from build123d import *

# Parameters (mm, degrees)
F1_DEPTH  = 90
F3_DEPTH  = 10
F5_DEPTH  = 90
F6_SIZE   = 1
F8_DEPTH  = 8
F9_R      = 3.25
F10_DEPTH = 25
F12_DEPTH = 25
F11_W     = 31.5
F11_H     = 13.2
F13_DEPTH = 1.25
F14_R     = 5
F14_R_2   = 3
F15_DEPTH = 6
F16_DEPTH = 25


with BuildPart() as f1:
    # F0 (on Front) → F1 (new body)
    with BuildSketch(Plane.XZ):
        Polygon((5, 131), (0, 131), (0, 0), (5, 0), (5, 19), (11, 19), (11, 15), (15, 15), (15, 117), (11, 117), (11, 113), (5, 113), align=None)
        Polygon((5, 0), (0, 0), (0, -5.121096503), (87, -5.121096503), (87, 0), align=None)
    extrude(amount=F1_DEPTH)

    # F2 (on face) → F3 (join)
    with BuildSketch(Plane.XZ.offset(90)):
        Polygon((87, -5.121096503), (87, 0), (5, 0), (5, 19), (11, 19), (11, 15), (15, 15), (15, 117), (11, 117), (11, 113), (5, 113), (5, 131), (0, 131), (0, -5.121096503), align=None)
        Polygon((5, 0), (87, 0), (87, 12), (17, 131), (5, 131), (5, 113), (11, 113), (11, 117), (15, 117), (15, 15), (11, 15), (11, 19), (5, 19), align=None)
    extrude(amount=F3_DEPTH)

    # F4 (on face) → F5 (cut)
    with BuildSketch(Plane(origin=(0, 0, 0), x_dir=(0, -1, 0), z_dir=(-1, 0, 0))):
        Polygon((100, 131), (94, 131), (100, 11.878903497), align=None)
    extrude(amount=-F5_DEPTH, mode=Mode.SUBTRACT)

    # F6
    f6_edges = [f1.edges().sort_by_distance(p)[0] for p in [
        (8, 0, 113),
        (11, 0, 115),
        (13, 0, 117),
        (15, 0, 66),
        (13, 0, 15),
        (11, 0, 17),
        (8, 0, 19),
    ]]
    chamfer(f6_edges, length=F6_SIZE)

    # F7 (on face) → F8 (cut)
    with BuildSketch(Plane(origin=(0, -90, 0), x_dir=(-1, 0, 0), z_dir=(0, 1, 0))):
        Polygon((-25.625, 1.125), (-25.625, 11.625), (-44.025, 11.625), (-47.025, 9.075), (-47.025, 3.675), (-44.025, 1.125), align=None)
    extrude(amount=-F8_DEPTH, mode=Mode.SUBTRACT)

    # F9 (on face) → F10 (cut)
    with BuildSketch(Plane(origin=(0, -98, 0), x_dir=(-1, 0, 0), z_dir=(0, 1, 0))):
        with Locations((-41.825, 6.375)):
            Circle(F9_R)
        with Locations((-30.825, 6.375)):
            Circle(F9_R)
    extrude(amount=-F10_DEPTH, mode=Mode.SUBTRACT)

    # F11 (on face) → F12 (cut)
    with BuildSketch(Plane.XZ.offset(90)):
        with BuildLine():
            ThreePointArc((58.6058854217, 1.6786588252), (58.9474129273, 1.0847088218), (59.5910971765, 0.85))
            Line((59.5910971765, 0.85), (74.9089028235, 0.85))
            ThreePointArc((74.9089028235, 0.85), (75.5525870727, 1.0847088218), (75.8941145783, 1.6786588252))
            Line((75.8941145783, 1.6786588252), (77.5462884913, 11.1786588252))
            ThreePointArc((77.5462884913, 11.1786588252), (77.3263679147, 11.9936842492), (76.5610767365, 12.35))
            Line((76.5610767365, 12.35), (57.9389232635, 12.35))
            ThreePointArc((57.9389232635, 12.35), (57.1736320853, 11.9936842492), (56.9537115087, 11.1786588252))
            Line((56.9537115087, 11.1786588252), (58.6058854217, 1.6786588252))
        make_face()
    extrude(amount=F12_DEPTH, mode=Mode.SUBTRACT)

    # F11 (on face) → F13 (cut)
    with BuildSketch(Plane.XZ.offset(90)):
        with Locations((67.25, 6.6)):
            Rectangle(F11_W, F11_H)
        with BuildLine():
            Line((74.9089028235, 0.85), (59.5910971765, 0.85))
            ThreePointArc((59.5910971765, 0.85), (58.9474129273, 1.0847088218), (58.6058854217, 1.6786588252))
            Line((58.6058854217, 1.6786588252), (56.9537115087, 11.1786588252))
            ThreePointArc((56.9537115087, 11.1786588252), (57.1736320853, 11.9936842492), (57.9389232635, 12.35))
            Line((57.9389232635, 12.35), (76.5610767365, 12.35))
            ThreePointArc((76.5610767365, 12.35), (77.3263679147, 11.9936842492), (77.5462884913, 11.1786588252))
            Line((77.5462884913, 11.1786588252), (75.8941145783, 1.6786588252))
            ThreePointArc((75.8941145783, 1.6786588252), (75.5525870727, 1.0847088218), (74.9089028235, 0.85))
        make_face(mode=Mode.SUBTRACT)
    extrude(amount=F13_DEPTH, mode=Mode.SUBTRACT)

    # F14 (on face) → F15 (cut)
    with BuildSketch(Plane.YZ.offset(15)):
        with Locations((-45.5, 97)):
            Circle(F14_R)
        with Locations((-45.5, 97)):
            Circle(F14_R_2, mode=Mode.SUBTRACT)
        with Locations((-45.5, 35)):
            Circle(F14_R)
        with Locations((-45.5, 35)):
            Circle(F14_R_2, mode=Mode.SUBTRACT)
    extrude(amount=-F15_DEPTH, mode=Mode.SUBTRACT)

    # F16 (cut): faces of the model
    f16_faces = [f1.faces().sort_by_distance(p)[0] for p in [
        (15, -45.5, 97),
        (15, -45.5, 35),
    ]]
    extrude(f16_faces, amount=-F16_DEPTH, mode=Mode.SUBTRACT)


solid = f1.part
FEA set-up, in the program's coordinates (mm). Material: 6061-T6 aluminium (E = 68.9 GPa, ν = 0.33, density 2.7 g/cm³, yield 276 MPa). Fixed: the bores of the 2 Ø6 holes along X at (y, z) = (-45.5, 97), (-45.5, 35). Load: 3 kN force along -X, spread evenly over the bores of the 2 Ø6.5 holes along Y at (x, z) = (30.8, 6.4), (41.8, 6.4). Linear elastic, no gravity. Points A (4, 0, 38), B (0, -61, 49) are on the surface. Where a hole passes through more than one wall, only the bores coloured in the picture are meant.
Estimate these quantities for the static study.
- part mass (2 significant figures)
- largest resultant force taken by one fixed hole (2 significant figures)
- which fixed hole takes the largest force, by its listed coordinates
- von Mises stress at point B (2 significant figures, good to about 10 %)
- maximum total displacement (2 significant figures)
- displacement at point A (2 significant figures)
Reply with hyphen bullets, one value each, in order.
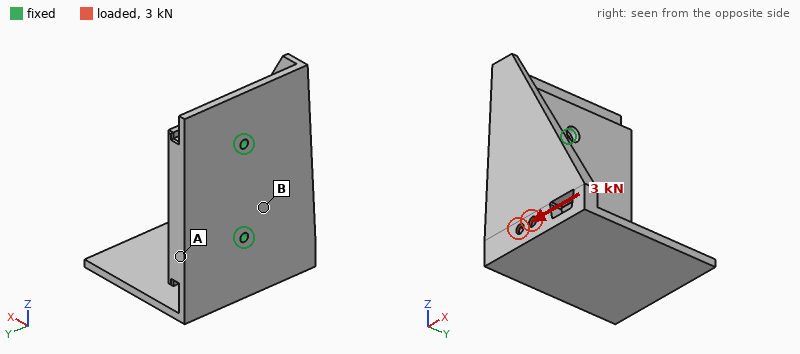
- 660 g
- 4.2 kN
- (-45.5, 35)
- 43 MPa
- 0.65 mm
- 0.13 mm
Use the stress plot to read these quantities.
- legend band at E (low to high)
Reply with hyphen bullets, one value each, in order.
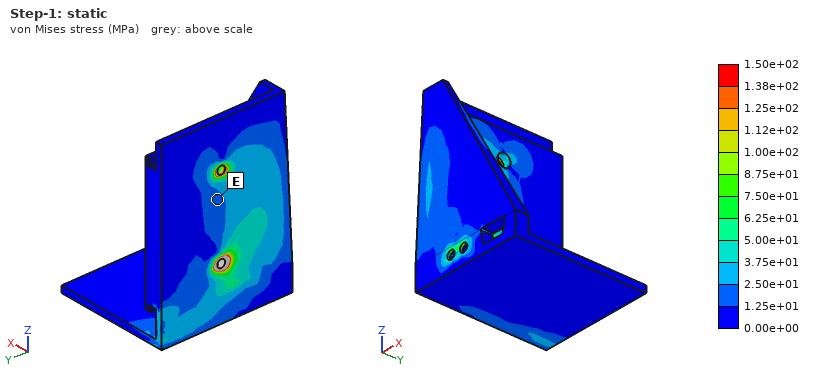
- 1.25e+01 to 2.50e+01 MPa
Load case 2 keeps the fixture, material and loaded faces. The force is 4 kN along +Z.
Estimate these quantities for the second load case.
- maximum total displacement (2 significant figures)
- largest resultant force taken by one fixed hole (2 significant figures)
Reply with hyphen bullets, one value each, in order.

- 0.17 mm
- 4.4 kN
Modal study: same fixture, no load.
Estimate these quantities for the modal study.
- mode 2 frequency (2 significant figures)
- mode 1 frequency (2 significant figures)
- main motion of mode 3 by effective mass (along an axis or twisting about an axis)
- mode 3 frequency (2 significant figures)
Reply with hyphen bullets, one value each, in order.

- 870 Hz
- 840 Hz
- along X
- 1900 Hz
